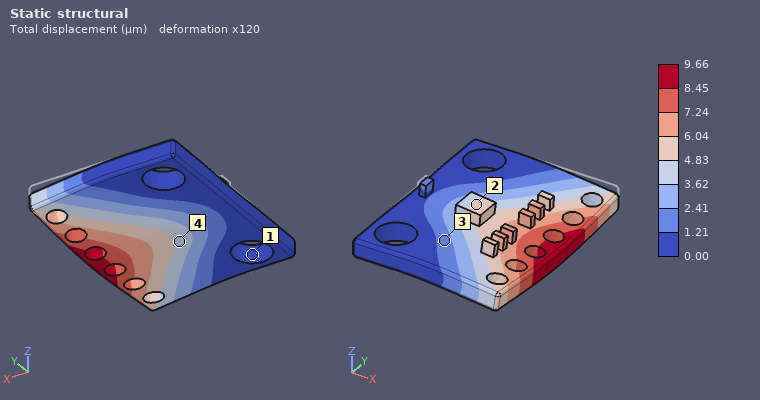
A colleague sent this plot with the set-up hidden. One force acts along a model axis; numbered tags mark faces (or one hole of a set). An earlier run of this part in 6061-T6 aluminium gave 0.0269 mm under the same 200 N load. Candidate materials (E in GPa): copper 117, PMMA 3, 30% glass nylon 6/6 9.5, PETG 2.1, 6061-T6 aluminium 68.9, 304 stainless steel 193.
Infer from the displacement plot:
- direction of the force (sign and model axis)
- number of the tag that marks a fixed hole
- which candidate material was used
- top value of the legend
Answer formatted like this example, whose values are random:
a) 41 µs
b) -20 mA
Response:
a) -Z
b) 1
c) 304 stainless steel
d) 9.66 µm
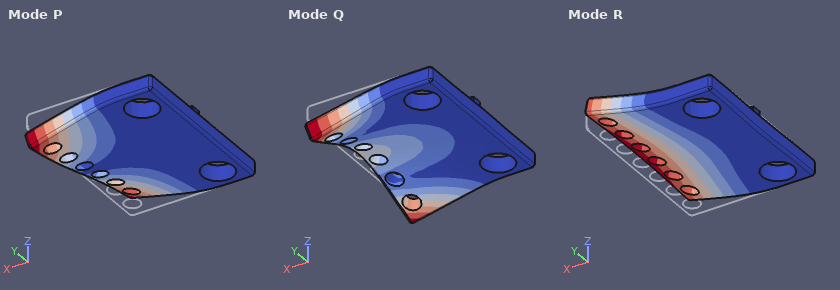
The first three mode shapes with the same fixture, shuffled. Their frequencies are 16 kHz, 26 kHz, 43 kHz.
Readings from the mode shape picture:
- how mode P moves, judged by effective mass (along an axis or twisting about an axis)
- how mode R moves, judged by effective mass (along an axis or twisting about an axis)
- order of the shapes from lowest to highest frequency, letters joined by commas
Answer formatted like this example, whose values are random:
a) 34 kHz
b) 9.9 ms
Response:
a) twisting about X
b) along Z
c) R, P, Q
